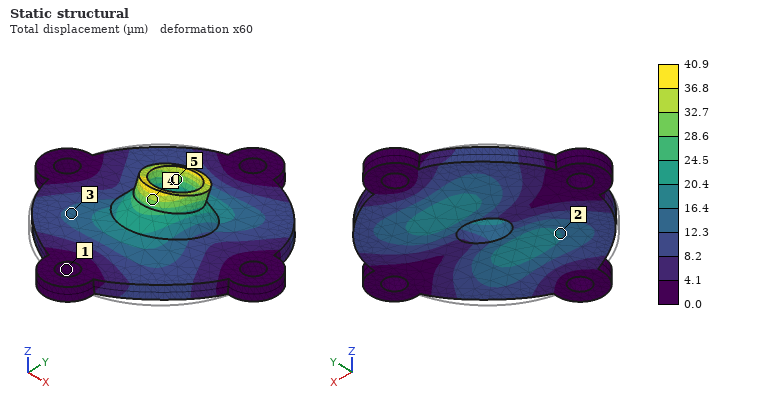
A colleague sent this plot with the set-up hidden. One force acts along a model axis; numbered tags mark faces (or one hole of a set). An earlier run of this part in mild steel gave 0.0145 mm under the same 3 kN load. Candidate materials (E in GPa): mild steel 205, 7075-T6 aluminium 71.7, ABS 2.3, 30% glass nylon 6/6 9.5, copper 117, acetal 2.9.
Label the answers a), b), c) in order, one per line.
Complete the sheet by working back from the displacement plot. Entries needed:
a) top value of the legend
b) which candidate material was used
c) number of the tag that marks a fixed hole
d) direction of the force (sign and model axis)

a) 40.9 µm
b) 7075-T6 aluminium
c) 1
d) +Y
